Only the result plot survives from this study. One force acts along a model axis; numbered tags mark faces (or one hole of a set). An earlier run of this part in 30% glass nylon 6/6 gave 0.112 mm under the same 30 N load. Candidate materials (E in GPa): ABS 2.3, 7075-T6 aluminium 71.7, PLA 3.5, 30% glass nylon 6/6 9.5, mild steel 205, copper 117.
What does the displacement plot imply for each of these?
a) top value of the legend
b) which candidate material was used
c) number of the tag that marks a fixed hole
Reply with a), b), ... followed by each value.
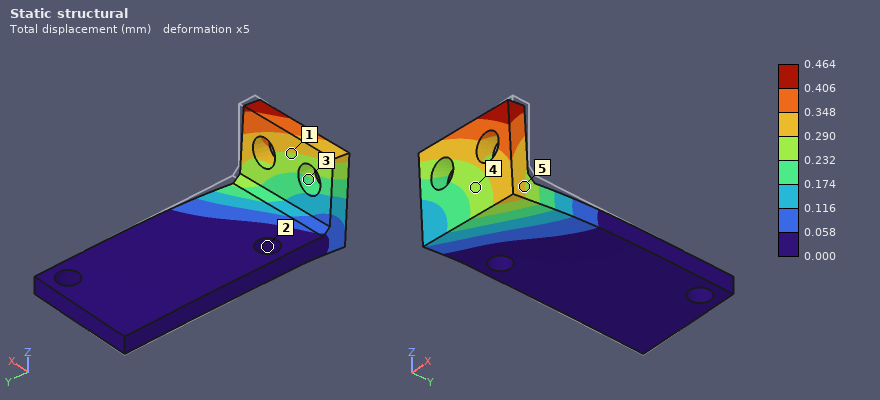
a) 0.464 mm
b) ABS
c) 2
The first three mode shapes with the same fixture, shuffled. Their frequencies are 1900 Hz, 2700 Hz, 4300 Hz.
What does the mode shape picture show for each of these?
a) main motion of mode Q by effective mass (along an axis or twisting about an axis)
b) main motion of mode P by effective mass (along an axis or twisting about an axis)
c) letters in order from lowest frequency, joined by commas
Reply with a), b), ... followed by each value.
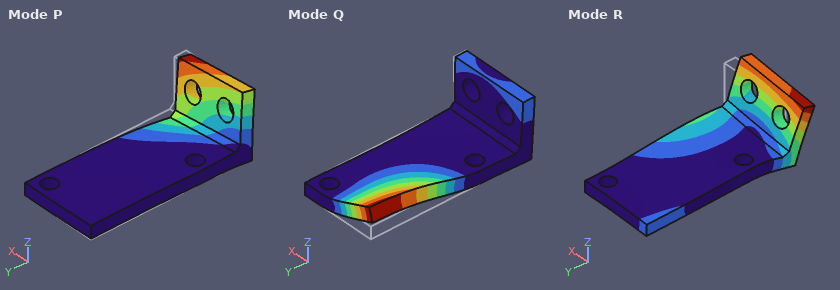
a) along Z
b) along Z
c) P, R, Q
